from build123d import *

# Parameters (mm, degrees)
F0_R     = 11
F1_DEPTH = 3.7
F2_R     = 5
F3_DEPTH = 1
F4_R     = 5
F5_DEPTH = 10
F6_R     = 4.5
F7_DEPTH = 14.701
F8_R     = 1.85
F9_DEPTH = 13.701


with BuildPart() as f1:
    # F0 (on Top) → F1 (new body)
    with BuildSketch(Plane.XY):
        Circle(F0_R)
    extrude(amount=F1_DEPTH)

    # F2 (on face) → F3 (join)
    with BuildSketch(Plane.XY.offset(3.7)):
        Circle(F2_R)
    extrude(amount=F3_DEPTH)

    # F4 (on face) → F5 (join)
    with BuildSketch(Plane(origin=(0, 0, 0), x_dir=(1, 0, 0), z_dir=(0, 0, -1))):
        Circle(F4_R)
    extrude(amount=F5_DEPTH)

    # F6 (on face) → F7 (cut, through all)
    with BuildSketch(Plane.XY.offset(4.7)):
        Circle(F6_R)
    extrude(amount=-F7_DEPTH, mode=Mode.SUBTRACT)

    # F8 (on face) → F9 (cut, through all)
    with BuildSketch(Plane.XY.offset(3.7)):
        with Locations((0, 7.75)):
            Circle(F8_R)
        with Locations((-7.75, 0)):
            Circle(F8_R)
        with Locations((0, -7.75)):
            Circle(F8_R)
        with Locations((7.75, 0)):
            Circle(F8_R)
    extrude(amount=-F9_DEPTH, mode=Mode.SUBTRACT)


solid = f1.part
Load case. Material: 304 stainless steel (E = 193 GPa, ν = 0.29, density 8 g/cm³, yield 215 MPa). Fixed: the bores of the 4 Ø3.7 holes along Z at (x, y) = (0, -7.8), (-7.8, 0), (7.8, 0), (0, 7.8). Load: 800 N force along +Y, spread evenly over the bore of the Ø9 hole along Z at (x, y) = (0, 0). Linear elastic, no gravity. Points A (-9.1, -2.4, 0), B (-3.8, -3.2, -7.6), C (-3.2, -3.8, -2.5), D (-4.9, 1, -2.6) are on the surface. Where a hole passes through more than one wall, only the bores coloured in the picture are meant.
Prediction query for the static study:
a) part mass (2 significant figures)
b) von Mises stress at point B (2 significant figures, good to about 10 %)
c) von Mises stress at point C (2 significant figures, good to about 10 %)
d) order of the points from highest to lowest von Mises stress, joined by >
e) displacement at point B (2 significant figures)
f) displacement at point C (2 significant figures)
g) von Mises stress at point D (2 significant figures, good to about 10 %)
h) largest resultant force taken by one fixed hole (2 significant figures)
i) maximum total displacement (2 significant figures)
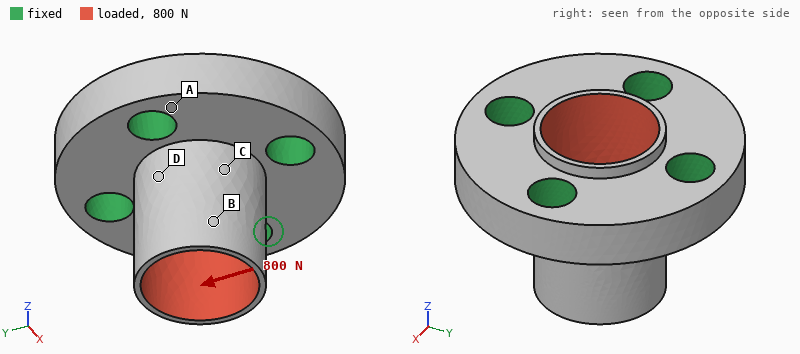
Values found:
9.4 g
26 MPa
65 MPa
D > C > B > A
7.5 µm
3.5 µm
84 MPa
330 N
9.2 µm
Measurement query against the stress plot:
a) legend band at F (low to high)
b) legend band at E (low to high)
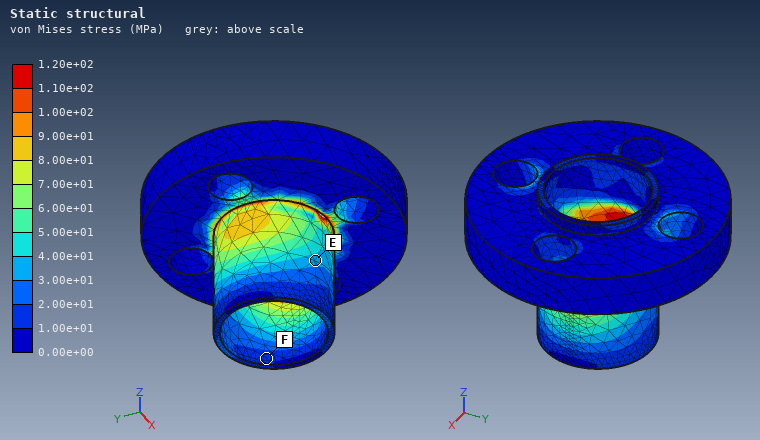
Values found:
1.00e+01 to 2.00e+01 MPa
3.00e+01 to 4.00e+01 MPa
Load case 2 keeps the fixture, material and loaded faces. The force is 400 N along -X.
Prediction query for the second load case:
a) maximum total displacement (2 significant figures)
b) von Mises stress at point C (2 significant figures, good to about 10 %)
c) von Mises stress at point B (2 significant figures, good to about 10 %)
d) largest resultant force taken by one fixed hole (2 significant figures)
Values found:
4.6 µm
36 MPa
12 MPa
170 N
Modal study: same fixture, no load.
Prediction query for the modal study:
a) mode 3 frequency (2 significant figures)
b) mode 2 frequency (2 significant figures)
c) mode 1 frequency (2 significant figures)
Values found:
41 kHz
26 kHz
25 kHz
